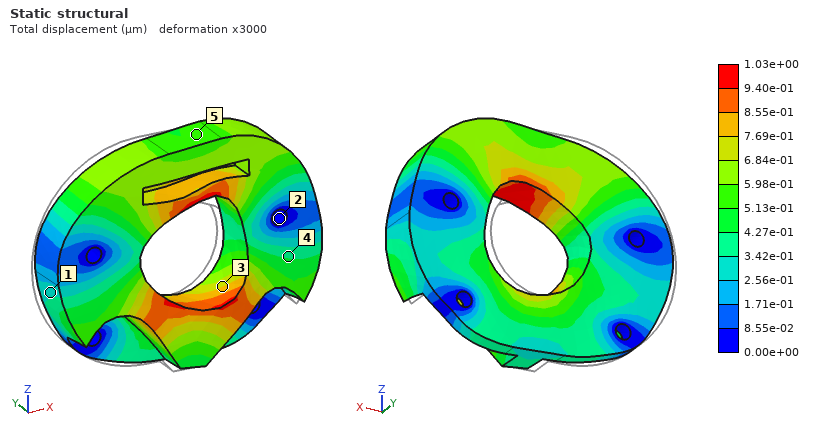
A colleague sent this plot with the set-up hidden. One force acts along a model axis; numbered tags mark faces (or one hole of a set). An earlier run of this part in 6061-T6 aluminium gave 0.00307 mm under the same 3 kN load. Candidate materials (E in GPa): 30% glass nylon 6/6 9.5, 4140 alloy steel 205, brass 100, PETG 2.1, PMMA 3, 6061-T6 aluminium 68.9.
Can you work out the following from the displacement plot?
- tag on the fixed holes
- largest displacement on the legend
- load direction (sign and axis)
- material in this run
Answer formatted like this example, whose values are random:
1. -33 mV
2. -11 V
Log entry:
1. 2
2. 1.03e+00 µm
3. +X
4. 4140 alloy steel
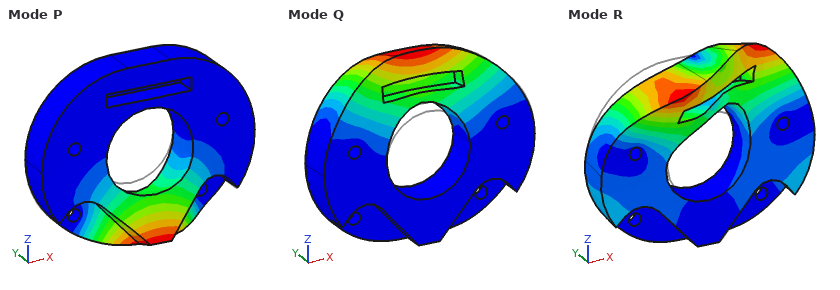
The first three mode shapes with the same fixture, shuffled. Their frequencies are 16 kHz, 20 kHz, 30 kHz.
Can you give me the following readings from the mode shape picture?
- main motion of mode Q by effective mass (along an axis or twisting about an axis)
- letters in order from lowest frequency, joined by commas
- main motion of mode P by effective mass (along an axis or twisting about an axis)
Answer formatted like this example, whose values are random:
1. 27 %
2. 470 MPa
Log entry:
1. along Y
2. Q, P, R
3. along Y
